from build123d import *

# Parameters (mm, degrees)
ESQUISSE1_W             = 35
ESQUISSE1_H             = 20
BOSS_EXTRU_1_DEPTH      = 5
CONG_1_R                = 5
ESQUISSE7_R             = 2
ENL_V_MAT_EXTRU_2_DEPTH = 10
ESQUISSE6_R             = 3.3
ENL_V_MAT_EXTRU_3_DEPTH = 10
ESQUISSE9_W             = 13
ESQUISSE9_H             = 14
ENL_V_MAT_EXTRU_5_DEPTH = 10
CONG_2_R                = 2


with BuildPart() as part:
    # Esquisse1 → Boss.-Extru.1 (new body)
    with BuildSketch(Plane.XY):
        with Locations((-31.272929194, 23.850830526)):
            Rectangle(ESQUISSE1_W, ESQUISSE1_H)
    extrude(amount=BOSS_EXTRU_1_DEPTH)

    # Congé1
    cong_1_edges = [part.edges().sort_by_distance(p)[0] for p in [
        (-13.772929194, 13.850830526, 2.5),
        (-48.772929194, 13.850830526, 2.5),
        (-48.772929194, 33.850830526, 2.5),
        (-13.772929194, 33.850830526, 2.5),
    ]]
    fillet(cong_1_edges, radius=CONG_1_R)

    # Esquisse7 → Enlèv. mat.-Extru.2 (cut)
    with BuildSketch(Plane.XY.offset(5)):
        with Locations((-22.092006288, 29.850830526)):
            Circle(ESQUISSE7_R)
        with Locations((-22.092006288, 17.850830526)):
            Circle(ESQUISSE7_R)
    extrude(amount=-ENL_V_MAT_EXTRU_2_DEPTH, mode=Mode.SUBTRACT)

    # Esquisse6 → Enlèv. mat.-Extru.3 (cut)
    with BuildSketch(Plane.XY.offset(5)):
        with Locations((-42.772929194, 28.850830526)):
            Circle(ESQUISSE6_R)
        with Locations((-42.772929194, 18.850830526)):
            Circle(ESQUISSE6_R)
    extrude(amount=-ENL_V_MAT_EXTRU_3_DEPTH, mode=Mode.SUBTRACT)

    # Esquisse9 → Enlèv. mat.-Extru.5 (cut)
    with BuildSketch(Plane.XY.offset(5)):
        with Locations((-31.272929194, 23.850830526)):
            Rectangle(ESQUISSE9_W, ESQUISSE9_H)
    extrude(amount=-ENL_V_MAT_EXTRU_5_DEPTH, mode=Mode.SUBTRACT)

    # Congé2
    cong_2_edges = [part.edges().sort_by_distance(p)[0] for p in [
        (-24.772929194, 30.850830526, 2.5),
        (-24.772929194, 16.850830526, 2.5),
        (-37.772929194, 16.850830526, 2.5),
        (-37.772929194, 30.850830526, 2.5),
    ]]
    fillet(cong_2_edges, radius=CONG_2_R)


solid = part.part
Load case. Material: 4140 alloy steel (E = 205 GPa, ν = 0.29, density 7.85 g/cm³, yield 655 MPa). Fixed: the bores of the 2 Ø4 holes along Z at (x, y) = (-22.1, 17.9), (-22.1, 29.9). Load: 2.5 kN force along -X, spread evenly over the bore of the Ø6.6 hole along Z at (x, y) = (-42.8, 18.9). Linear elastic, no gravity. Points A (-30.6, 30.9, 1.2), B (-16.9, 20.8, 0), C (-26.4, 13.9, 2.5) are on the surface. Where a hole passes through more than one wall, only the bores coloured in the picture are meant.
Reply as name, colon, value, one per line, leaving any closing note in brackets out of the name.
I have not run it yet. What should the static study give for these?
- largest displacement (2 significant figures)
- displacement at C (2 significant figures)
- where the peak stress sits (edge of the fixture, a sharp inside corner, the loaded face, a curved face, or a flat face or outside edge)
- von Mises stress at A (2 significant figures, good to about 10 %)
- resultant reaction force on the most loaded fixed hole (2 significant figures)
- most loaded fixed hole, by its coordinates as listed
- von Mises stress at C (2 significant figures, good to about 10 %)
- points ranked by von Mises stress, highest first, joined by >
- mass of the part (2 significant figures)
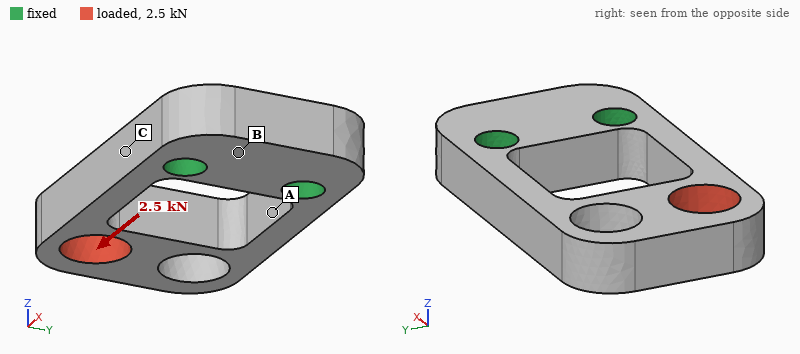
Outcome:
largest displacement: 21 µm
displacement at C: 4.9 µm
where the peak stress sits: the loaded face
von Mises stress at A: 64 MPa
resultant reaction force on the most loaded fixed hole: 2.0 kN
most loaded fixed hole, by its coordinates as listed: (-22.1, 17.9)
von Mises stress at C: 140 MPa
points ranked by von Mises stress, highest first, joined by >: C > A > B
mass of the part: 16 g
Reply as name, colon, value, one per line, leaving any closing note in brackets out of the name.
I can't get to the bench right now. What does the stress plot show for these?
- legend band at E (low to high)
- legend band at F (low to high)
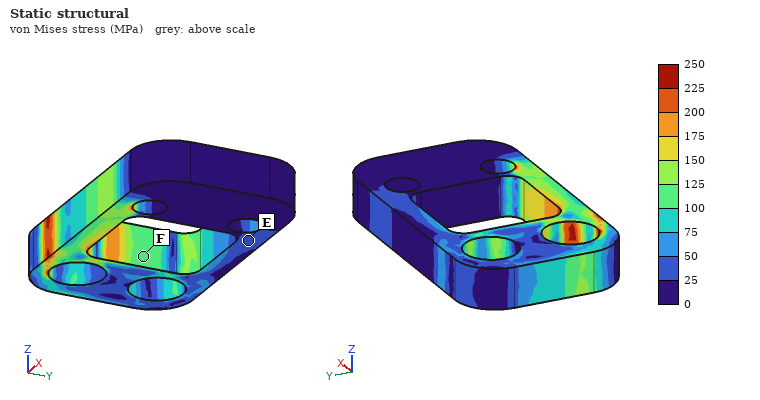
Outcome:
legend band at E: 25 to 50 MPa
legend band at F: 100 to 125 MPa
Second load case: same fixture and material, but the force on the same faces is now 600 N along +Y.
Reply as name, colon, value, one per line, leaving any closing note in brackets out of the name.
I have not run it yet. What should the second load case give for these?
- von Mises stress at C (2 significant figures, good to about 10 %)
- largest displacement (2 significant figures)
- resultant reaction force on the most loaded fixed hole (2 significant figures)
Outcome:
von Mises stress at C: 230 MPa
largest displacement: 54 µm
resultant reaction force on the most loaded fixed hole: 550 N
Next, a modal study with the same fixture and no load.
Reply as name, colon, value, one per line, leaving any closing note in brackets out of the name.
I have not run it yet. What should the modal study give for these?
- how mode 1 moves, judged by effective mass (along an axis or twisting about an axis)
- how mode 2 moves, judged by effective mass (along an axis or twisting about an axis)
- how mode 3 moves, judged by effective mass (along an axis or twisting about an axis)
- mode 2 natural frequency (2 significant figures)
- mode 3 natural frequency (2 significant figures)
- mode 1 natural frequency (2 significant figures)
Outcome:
how mode 1 moves, judged by effective mass: along Z
how mode 2 moves, judged by effective mass: along Y
how mode 3 moves, judged by effective mass: twisting about X
mode 2 natural frequency: 6900 Hz
mode 3 natural frequency: 11 kHz
mode 1 natural frequency: 4300 Hz
